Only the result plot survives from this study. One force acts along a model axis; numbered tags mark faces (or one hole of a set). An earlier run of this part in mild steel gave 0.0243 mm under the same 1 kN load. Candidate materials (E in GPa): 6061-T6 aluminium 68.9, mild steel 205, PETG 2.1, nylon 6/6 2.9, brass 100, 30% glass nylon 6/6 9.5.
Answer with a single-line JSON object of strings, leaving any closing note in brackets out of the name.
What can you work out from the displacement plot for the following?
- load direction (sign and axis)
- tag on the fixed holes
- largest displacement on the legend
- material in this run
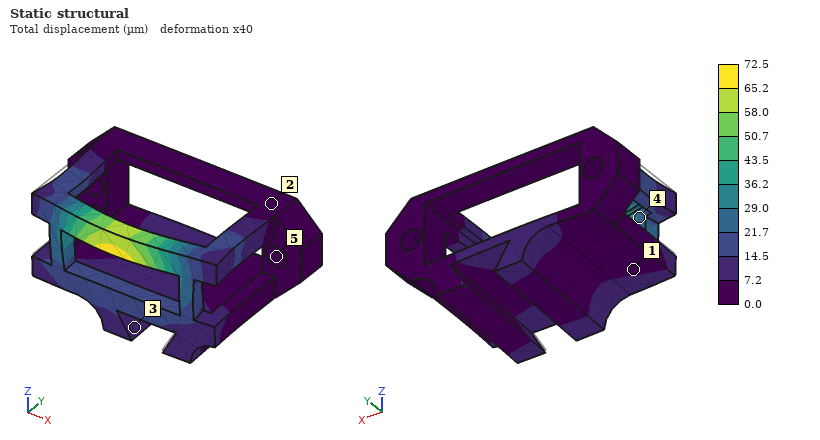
{"load direction": "-Y", "tag on the fixed holes": "5", "largest displacement on the legend": "72.5 µm", "material in this run": "6061-T6 aluminium"}
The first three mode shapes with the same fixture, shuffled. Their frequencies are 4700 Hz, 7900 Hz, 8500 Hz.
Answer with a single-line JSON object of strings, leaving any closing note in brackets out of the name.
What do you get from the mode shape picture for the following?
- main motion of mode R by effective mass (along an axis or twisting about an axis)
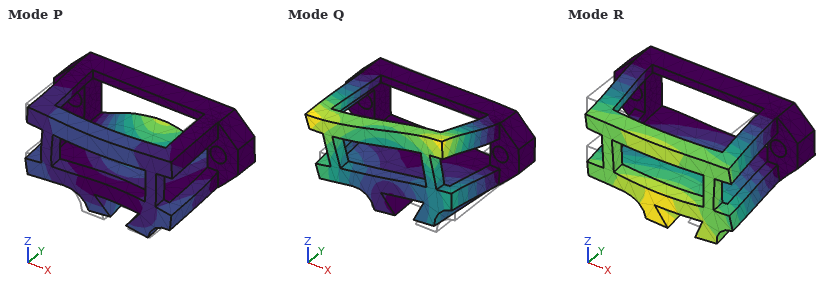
{"main motion of mode R by effective mass": "along Z"}
